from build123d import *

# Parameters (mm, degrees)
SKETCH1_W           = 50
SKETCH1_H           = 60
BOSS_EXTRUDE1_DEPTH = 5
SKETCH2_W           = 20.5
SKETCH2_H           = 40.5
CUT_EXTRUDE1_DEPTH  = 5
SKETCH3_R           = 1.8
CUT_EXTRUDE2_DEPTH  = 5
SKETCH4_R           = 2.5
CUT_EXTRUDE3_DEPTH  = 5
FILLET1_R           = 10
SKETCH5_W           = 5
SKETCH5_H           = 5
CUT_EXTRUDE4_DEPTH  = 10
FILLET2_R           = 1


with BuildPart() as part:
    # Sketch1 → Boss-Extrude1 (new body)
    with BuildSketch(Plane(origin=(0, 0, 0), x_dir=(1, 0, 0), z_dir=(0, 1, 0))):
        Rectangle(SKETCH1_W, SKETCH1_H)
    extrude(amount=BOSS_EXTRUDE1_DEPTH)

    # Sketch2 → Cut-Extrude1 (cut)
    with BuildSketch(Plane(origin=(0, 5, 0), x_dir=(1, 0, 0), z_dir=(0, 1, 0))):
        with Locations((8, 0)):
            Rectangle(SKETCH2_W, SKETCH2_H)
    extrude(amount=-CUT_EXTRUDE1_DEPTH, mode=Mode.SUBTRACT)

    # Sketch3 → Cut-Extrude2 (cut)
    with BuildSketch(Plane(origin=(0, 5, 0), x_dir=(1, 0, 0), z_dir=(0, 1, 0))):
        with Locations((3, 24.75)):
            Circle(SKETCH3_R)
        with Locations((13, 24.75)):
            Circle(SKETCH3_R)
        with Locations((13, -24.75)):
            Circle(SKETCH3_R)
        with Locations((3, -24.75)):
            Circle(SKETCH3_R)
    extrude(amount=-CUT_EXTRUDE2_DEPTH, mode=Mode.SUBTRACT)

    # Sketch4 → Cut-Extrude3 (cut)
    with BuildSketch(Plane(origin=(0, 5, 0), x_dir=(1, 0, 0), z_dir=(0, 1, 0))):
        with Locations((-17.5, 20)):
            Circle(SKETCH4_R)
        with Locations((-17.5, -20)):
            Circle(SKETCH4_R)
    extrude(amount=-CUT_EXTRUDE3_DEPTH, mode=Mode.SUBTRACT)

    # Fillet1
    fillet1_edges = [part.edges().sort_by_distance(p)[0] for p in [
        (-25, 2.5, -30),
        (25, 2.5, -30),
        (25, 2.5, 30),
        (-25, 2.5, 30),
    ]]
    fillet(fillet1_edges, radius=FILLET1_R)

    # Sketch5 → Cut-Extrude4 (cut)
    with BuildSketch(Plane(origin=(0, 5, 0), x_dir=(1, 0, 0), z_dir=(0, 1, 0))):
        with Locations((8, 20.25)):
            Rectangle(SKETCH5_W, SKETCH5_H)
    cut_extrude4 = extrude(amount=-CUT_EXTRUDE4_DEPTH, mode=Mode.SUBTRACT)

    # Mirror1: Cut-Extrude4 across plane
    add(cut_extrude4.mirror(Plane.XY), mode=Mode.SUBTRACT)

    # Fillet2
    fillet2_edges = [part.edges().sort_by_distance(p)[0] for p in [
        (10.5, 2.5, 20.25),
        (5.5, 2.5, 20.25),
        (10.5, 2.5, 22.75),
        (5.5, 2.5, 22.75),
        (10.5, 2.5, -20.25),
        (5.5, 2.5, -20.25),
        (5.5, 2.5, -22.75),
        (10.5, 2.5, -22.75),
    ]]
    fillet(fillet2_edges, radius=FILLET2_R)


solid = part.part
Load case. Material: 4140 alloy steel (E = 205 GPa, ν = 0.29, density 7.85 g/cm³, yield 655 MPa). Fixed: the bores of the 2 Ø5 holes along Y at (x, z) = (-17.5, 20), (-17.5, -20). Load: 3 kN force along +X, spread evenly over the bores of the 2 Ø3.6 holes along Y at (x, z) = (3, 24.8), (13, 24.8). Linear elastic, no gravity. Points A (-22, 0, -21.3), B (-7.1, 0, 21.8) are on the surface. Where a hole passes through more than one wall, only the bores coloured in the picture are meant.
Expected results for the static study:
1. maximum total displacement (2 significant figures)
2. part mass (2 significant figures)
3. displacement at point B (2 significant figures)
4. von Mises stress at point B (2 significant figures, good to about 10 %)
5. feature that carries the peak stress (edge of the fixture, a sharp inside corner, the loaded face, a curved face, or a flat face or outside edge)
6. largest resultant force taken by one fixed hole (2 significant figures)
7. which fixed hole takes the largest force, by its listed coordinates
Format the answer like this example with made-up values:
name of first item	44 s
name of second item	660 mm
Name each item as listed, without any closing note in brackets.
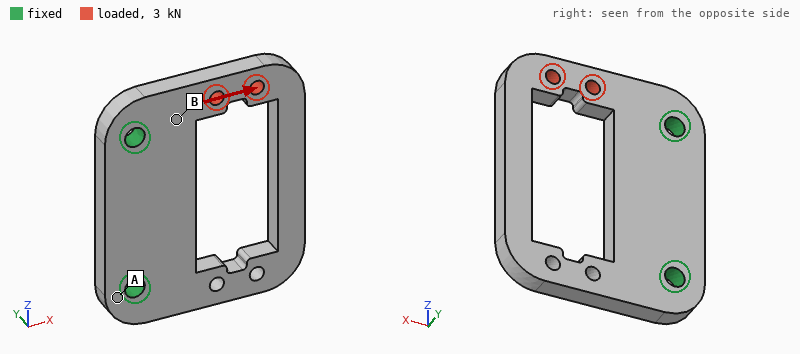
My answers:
maximum total displacement	14 µm
part mass	78 g
displacement at point B	3.1 µm
von Mises stress at point B	56 MPa
feature that carries the peak stress	a curved face
largest resultant force taken by one fixed hole	3.2 kN
which fixed hole takes the largest force, by its listed coordinates	(-17.5, 20)
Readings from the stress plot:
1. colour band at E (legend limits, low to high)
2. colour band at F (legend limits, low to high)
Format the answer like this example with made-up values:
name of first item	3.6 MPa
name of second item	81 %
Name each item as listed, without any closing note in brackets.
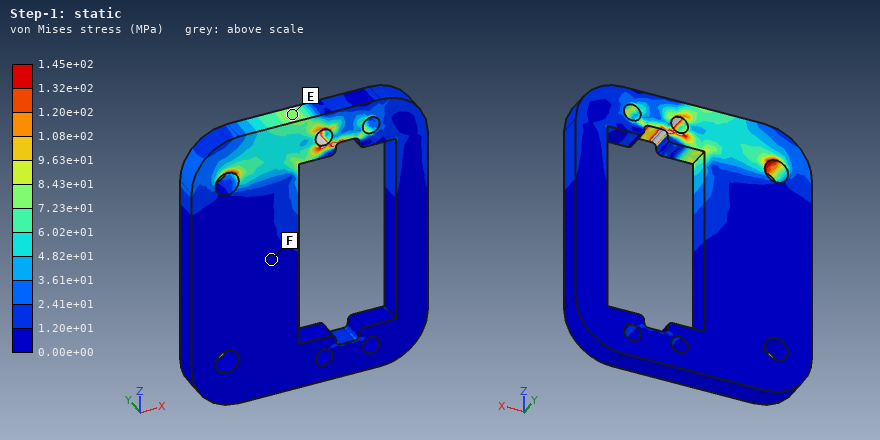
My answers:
colour band at E	7.23e+01 to 8.43e+01 MPa
colour band at F	0.00e+00 to 1.20e+01 MPa
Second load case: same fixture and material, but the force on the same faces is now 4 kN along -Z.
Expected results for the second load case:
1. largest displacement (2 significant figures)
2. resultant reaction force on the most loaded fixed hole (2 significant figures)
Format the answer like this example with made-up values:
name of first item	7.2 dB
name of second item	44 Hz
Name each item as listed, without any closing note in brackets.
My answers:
largest displacement	80 µm
resultant reaction force on the most loaded fixed hole	2.9 kN
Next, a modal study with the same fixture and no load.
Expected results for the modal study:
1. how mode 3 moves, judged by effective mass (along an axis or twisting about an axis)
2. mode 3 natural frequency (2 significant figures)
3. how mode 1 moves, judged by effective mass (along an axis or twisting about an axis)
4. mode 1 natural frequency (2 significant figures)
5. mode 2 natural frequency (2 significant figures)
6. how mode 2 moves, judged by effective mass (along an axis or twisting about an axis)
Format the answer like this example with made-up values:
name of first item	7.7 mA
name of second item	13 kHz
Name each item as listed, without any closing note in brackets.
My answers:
how mode 3 moves, judged by effective mass	along Z
mode 3 natural frequency	5800 Hz
how mode 1 moves, judged by effective mass	along Y
mode 1 natural frequency	1900 Hz
mode 2 natural frequency	3700 Hz
how mode 2 moves, judged by effective mass	twisting about X
